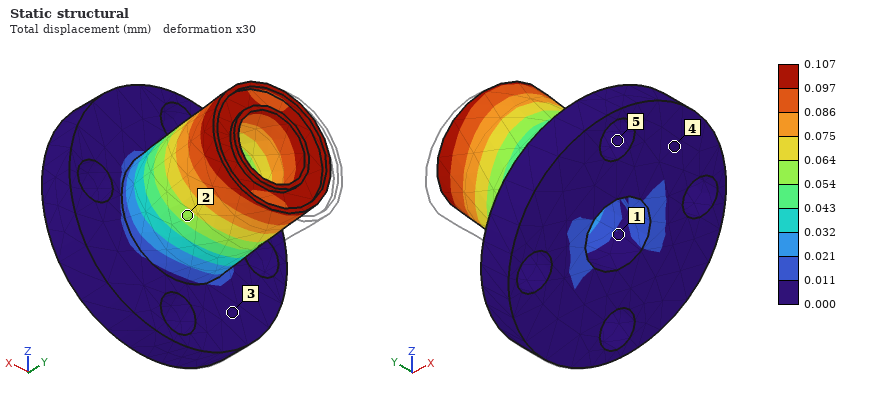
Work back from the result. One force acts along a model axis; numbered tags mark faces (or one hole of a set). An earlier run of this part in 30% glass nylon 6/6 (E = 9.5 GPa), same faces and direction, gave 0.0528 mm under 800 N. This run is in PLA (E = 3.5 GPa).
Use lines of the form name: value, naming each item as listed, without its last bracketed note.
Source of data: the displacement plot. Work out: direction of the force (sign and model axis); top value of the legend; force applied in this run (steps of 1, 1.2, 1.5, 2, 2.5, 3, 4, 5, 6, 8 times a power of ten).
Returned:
direction of the force: +X
top value of the legend: 0.107 mm
force applied in this run: 600 N
